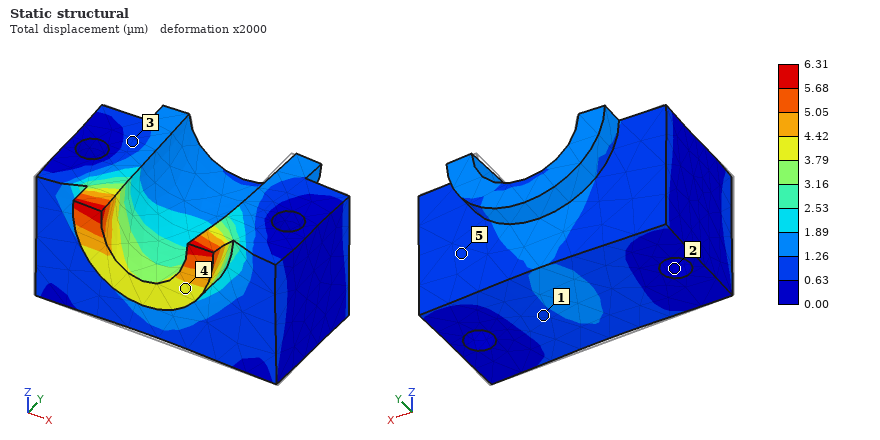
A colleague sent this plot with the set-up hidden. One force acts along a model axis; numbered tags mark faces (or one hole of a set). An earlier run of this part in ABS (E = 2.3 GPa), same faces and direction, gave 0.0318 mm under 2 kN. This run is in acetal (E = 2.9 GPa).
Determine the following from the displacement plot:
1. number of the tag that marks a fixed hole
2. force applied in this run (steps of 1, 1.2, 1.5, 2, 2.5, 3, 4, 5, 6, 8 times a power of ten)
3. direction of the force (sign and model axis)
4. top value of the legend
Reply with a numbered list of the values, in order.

1. 2
2. 500 N
3. +Y
4. 6.31 µm
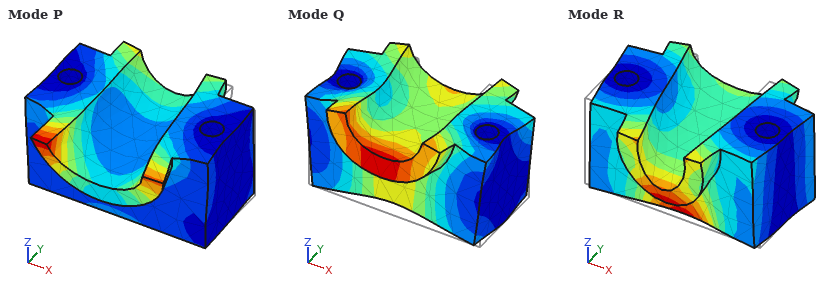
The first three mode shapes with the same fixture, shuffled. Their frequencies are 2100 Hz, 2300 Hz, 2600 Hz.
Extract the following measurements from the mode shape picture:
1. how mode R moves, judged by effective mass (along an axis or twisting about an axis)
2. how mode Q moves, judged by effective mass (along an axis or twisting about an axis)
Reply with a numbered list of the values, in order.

1. along Y
2. along Z
